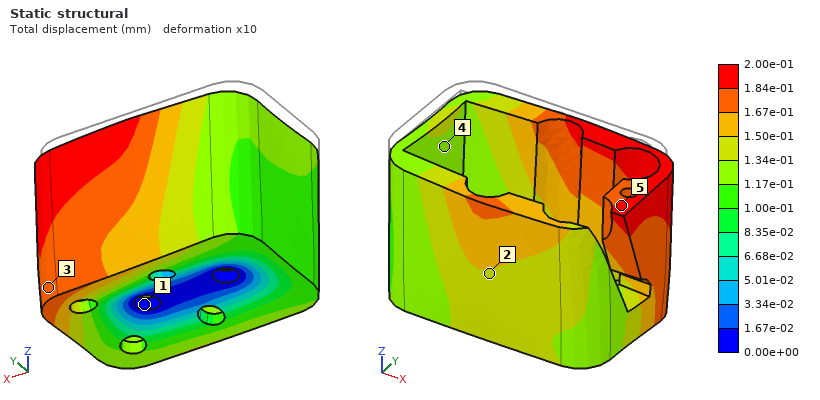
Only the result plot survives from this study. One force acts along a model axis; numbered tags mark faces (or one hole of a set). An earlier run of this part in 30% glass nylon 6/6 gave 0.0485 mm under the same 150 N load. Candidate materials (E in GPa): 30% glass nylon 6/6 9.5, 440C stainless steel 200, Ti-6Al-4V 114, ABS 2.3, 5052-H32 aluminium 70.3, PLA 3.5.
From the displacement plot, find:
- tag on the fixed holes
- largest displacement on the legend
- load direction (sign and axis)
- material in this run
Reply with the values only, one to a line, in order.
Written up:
1
2.00e-01 mm
-Z
ABS
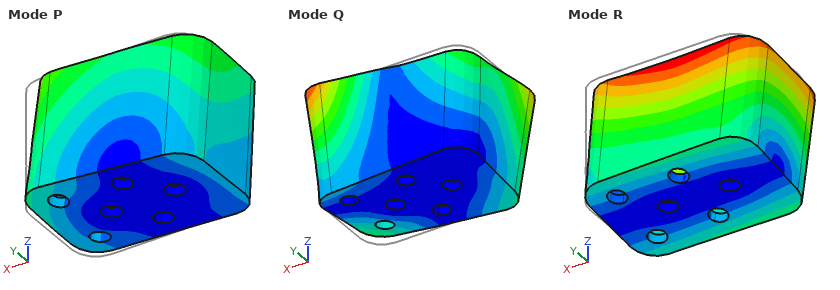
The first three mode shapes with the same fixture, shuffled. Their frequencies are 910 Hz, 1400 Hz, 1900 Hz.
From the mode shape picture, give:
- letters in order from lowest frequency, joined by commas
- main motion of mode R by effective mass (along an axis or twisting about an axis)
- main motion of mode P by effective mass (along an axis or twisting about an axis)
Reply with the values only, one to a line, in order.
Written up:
R, P, Q
along Y
along X
